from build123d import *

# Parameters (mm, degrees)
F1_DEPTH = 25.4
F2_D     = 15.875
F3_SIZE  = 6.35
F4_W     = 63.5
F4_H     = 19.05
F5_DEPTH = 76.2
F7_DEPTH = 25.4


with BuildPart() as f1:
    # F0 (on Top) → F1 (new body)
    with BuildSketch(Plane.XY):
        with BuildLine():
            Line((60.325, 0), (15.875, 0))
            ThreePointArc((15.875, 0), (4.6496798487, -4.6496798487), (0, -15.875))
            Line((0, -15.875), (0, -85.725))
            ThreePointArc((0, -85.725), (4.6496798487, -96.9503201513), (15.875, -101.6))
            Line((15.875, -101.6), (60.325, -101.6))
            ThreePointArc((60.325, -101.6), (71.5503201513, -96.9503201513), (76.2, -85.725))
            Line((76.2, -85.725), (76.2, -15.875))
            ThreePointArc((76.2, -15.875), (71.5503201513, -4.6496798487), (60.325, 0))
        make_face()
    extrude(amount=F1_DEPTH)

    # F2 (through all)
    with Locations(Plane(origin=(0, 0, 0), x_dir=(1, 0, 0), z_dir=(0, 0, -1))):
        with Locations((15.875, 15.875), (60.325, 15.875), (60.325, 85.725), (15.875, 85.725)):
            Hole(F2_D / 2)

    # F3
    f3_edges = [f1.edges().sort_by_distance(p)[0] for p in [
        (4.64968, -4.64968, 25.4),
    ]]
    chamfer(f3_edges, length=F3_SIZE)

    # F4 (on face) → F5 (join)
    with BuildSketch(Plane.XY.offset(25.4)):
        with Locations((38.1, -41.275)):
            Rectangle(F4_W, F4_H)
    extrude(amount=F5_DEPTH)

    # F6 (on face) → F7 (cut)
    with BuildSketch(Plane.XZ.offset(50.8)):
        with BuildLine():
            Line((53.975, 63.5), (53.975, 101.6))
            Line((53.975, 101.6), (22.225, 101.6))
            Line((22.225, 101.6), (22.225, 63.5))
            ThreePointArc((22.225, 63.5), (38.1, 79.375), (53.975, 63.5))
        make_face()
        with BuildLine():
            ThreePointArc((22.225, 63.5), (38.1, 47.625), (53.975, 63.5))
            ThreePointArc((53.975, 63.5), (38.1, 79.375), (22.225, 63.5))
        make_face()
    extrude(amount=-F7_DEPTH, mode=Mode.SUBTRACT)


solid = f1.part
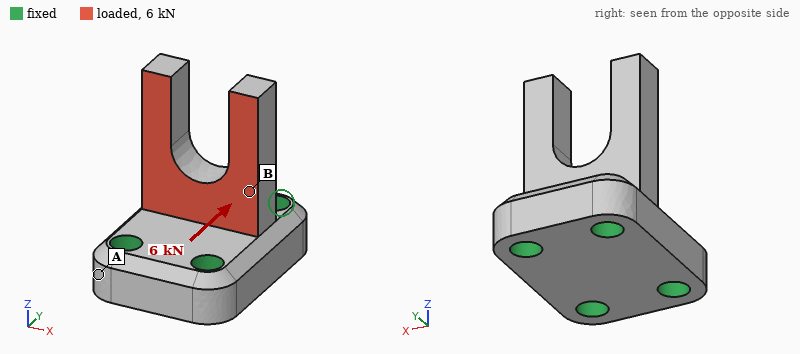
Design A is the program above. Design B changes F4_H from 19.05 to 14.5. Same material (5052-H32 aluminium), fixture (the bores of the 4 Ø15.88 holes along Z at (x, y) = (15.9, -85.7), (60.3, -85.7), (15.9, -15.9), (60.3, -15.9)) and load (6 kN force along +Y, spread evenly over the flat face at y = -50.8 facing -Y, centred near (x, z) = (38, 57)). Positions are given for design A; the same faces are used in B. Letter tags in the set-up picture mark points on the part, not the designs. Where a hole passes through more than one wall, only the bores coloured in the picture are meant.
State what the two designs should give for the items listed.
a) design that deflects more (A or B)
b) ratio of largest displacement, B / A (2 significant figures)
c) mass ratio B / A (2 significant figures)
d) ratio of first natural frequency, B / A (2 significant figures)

B
2.0
0.93
0.80
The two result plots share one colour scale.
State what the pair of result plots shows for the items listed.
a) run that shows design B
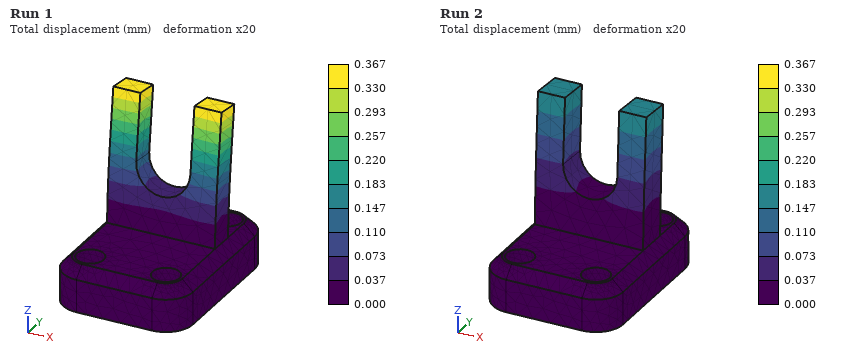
Run 1
